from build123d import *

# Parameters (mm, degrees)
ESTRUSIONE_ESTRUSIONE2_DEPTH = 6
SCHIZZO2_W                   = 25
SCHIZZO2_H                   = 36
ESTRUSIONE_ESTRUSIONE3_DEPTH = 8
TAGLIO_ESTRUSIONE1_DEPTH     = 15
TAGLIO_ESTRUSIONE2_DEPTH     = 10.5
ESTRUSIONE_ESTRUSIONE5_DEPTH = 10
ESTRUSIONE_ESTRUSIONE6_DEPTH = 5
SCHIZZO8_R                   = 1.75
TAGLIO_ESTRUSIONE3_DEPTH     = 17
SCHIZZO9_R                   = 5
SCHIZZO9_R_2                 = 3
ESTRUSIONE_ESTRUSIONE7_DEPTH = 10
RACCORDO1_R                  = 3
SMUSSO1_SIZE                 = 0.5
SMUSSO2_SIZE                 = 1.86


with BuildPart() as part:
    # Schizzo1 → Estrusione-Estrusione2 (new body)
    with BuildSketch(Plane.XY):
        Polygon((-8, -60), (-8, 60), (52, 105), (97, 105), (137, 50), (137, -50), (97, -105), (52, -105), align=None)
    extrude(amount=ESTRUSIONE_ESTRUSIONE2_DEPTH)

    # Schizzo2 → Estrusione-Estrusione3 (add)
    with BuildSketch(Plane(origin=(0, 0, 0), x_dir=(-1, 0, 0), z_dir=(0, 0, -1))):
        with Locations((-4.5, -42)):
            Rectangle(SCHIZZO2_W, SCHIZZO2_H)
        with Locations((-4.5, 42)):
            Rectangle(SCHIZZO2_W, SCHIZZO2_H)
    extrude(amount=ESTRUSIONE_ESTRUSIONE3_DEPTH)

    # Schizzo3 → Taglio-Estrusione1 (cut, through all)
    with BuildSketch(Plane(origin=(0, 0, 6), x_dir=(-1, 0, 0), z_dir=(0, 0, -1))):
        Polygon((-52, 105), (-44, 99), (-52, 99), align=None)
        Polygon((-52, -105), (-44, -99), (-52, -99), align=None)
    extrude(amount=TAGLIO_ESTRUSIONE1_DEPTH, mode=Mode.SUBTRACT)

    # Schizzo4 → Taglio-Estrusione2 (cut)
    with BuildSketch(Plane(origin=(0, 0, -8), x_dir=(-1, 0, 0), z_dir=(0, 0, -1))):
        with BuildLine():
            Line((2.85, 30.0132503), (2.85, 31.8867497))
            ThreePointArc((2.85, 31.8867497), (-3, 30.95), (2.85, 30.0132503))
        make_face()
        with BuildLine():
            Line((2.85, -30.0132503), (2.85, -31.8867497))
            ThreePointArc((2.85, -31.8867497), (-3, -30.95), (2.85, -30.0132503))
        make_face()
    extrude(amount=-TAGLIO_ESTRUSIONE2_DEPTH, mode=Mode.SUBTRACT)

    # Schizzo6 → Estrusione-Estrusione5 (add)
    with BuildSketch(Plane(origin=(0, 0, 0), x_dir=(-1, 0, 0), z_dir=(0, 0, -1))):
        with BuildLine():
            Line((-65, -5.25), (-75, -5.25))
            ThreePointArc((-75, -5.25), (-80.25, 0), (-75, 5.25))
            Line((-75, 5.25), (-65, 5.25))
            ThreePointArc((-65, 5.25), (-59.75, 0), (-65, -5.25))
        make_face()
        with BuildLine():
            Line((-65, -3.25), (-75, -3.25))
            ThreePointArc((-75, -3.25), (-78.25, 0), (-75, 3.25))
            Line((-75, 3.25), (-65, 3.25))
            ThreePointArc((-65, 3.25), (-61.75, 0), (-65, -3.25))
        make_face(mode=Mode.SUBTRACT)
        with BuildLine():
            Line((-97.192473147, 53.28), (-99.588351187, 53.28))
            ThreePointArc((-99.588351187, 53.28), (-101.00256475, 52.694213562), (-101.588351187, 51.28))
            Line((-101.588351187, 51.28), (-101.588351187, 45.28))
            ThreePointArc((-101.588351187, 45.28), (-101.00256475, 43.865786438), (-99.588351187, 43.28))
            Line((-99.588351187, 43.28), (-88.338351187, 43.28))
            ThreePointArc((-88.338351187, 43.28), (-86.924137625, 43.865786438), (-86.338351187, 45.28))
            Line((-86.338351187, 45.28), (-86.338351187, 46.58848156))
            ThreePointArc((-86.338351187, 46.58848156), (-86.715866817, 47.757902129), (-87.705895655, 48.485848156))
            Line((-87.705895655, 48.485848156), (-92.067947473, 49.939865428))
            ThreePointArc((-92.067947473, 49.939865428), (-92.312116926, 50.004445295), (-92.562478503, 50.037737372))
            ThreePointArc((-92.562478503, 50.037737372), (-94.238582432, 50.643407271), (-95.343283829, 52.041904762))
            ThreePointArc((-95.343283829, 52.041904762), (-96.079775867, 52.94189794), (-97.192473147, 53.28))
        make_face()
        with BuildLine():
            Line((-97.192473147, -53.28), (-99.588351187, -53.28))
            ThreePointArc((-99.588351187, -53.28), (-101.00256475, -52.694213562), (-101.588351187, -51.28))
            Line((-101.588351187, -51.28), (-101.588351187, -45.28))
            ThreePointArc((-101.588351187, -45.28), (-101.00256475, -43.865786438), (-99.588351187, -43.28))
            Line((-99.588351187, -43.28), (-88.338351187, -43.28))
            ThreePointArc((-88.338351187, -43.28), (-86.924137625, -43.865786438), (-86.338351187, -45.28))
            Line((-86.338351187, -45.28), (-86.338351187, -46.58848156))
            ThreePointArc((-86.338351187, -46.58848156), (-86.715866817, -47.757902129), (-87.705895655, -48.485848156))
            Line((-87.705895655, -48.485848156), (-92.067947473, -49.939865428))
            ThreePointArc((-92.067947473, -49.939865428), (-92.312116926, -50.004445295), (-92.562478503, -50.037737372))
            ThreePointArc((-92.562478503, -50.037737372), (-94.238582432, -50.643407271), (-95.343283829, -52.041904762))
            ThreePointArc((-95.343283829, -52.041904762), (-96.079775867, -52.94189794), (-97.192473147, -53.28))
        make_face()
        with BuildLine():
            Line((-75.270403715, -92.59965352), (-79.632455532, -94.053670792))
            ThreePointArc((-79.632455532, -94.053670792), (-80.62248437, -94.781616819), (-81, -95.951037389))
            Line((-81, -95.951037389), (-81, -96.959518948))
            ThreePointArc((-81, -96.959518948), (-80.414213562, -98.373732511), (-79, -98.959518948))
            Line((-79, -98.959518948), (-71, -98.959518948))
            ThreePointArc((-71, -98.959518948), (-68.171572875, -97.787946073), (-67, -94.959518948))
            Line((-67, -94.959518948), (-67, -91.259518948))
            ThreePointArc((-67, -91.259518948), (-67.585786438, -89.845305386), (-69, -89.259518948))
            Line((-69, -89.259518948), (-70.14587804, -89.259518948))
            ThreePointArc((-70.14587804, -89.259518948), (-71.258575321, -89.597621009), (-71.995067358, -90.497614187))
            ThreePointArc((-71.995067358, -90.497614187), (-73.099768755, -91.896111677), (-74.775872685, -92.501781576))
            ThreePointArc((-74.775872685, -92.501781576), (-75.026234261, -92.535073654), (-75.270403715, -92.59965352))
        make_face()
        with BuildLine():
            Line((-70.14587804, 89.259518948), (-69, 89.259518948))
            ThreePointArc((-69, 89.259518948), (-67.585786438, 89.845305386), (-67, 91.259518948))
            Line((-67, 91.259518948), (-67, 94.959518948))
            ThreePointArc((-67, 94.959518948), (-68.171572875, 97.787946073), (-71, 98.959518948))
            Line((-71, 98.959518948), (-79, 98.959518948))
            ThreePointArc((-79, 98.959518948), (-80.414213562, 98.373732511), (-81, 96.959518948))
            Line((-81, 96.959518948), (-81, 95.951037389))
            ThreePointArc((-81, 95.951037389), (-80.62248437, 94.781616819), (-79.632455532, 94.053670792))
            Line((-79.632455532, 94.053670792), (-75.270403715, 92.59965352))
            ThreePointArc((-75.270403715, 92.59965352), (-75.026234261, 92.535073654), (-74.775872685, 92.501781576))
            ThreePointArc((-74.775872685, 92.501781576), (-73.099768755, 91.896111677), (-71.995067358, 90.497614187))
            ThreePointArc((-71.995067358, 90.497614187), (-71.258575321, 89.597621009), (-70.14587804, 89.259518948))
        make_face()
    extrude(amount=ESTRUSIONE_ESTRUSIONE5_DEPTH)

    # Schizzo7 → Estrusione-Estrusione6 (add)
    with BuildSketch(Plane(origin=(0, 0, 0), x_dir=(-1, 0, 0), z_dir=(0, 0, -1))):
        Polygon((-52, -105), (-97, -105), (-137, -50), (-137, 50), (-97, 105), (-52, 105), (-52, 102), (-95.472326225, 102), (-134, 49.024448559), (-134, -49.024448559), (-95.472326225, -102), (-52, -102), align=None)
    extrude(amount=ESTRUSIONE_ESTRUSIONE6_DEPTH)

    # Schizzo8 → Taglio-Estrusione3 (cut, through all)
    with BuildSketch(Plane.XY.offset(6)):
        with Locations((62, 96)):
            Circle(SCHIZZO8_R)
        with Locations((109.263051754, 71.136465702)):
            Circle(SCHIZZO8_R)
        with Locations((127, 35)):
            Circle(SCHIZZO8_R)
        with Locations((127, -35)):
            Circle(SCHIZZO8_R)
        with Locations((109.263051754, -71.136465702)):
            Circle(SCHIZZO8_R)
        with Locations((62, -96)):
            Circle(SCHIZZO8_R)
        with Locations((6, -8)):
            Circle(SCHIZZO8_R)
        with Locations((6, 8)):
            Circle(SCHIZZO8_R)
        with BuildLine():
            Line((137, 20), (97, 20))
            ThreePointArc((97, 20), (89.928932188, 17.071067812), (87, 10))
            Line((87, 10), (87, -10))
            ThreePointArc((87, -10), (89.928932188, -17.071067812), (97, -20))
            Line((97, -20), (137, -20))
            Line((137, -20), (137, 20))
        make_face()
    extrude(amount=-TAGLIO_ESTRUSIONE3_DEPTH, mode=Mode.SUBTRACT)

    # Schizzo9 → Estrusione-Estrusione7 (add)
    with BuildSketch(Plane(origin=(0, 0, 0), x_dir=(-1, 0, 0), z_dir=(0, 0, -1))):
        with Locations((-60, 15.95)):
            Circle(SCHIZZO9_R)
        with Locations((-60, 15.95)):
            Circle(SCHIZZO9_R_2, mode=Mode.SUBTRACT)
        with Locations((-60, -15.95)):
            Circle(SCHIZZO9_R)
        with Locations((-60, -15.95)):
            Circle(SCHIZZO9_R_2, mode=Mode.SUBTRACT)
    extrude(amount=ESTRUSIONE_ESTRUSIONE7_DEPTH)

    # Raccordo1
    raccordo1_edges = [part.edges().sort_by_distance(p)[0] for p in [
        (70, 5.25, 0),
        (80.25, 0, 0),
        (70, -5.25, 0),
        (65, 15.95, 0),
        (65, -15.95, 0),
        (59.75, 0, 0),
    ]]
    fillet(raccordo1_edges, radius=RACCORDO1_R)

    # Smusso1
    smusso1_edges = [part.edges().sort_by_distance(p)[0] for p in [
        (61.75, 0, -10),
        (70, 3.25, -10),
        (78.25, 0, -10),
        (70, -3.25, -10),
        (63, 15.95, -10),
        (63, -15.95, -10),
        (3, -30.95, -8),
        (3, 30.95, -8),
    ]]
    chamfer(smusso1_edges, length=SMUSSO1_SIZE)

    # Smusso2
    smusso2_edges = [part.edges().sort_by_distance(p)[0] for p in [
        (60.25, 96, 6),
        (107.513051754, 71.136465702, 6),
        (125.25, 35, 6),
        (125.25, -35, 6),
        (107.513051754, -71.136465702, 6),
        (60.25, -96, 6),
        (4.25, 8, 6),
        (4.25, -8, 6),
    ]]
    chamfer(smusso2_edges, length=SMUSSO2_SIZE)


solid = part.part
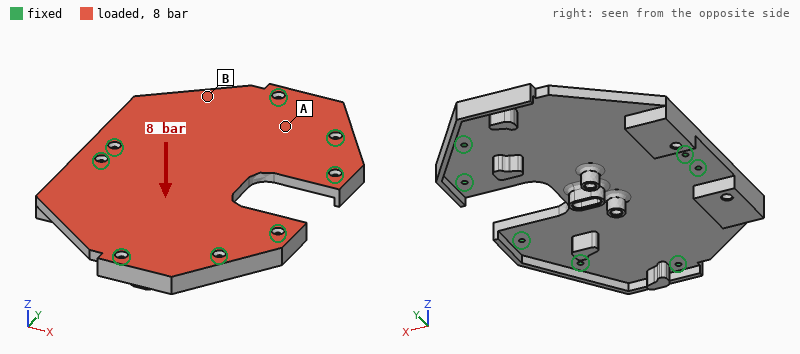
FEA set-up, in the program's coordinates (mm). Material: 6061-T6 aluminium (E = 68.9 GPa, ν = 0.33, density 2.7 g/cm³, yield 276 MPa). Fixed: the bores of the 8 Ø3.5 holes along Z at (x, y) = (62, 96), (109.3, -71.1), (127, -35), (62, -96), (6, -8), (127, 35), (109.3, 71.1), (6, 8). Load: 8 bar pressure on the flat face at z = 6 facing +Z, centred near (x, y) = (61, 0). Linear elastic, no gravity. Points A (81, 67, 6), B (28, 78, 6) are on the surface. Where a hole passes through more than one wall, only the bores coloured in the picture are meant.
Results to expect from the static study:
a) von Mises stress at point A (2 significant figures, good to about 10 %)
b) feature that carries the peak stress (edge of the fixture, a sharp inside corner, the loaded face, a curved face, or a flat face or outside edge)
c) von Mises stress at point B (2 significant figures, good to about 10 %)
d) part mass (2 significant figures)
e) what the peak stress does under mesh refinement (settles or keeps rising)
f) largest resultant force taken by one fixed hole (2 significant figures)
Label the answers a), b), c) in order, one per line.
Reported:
a) 34 MPa
b) edge of the fixture
c) 87 MPa
d) 450 g
e) keeps rising
f) 3.4 kN
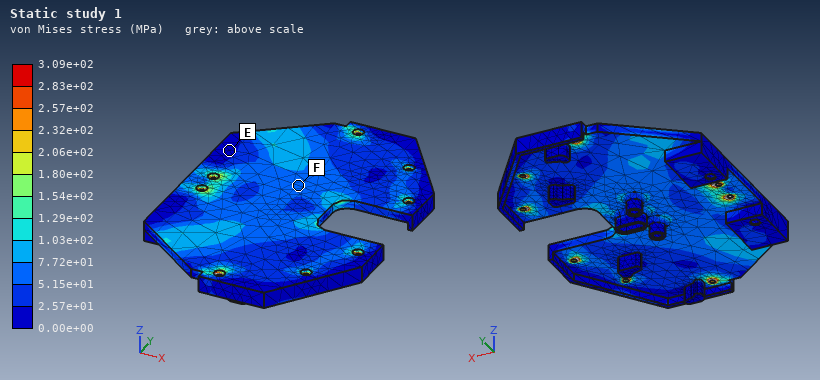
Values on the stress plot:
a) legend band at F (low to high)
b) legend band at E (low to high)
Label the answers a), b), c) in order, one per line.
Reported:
a) 5.15e+01 to 7.72e+01 MPa
b) 0.00e+00 to 2.57e+01 MPa
